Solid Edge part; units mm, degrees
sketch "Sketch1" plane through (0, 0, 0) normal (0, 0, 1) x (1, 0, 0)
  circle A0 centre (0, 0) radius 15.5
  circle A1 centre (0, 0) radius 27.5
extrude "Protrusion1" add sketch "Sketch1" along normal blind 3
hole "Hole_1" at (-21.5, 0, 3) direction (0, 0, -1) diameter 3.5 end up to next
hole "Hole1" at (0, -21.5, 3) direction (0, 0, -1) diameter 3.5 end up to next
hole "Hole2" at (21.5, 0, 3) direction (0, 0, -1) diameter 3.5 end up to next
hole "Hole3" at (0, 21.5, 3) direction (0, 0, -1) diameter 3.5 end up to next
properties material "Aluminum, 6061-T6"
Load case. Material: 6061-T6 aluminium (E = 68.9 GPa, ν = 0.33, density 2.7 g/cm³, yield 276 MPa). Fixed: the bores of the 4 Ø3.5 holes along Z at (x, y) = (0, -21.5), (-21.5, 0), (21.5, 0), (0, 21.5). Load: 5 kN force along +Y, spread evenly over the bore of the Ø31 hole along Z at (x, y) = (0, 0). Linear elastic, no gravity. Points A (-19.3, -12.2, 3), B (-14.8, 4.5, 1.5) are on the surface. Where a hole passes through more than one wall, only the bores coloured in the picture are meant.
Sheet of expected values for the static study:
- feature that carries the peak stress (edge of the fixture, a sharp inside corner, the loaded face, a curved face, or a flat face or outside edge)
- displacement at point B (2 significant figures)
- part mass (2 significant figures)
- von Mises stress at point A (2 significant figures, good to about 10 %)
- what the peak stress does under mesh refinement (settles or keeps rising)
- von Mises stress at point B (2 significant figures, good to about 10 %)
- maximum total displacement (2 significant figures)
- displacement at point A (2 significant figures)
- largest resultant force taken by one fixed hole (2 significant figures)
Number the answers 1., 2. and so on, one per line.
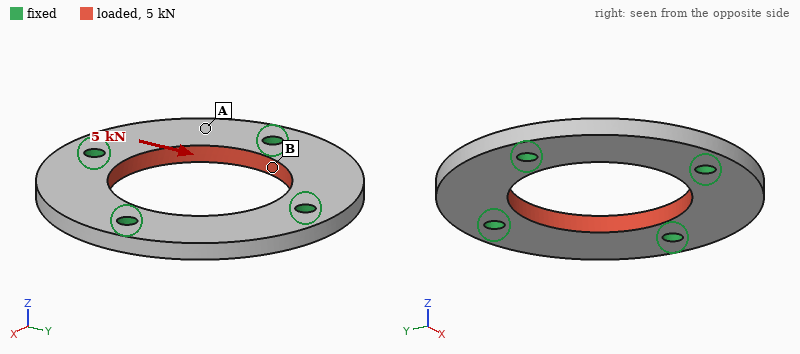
1. edge of the fixture
2. 6.8 µm
3. 13 g
4. 15 MPa
5. keeps rising
6. 31 MPa
7. 8.2 µm
8. 5.4 µm
9. 1.4 kN
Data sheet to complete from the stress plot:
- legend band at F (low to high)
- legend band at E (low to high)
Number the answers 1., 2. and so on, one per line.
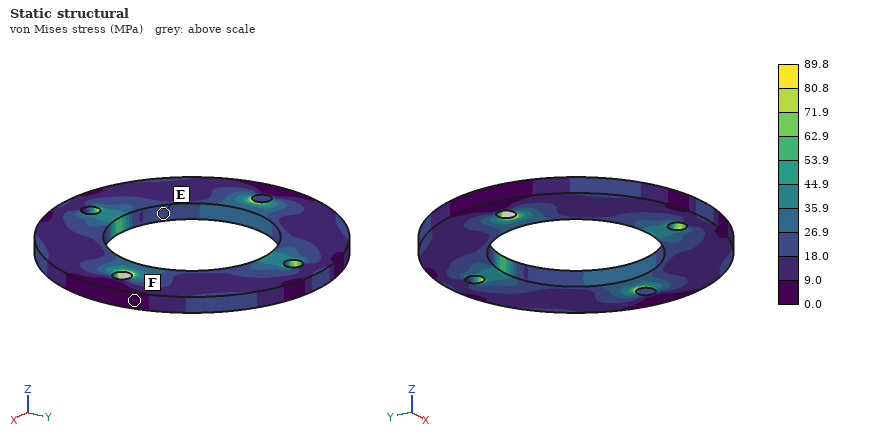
1. 0.0 to 9.0 MPa
2. 18.0 to 26.9 MPa
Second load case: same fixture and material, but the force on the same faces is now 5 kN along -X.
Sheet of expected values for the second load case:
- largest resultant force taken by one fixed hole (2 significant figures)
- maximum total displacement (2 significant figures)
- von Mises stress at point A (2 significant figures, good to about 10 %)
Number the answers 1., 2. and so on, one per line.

1. 1.4 kN
2. 8.2 µm
3. 14 MPa
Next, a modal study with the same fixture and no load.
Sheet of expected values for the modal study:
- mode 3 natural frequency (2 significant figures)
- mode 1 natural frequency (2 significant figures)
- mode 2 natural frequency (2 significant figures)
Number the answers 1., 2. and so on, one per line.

1. 12 kHz
2. 12 kHz
3. 12 kHz
